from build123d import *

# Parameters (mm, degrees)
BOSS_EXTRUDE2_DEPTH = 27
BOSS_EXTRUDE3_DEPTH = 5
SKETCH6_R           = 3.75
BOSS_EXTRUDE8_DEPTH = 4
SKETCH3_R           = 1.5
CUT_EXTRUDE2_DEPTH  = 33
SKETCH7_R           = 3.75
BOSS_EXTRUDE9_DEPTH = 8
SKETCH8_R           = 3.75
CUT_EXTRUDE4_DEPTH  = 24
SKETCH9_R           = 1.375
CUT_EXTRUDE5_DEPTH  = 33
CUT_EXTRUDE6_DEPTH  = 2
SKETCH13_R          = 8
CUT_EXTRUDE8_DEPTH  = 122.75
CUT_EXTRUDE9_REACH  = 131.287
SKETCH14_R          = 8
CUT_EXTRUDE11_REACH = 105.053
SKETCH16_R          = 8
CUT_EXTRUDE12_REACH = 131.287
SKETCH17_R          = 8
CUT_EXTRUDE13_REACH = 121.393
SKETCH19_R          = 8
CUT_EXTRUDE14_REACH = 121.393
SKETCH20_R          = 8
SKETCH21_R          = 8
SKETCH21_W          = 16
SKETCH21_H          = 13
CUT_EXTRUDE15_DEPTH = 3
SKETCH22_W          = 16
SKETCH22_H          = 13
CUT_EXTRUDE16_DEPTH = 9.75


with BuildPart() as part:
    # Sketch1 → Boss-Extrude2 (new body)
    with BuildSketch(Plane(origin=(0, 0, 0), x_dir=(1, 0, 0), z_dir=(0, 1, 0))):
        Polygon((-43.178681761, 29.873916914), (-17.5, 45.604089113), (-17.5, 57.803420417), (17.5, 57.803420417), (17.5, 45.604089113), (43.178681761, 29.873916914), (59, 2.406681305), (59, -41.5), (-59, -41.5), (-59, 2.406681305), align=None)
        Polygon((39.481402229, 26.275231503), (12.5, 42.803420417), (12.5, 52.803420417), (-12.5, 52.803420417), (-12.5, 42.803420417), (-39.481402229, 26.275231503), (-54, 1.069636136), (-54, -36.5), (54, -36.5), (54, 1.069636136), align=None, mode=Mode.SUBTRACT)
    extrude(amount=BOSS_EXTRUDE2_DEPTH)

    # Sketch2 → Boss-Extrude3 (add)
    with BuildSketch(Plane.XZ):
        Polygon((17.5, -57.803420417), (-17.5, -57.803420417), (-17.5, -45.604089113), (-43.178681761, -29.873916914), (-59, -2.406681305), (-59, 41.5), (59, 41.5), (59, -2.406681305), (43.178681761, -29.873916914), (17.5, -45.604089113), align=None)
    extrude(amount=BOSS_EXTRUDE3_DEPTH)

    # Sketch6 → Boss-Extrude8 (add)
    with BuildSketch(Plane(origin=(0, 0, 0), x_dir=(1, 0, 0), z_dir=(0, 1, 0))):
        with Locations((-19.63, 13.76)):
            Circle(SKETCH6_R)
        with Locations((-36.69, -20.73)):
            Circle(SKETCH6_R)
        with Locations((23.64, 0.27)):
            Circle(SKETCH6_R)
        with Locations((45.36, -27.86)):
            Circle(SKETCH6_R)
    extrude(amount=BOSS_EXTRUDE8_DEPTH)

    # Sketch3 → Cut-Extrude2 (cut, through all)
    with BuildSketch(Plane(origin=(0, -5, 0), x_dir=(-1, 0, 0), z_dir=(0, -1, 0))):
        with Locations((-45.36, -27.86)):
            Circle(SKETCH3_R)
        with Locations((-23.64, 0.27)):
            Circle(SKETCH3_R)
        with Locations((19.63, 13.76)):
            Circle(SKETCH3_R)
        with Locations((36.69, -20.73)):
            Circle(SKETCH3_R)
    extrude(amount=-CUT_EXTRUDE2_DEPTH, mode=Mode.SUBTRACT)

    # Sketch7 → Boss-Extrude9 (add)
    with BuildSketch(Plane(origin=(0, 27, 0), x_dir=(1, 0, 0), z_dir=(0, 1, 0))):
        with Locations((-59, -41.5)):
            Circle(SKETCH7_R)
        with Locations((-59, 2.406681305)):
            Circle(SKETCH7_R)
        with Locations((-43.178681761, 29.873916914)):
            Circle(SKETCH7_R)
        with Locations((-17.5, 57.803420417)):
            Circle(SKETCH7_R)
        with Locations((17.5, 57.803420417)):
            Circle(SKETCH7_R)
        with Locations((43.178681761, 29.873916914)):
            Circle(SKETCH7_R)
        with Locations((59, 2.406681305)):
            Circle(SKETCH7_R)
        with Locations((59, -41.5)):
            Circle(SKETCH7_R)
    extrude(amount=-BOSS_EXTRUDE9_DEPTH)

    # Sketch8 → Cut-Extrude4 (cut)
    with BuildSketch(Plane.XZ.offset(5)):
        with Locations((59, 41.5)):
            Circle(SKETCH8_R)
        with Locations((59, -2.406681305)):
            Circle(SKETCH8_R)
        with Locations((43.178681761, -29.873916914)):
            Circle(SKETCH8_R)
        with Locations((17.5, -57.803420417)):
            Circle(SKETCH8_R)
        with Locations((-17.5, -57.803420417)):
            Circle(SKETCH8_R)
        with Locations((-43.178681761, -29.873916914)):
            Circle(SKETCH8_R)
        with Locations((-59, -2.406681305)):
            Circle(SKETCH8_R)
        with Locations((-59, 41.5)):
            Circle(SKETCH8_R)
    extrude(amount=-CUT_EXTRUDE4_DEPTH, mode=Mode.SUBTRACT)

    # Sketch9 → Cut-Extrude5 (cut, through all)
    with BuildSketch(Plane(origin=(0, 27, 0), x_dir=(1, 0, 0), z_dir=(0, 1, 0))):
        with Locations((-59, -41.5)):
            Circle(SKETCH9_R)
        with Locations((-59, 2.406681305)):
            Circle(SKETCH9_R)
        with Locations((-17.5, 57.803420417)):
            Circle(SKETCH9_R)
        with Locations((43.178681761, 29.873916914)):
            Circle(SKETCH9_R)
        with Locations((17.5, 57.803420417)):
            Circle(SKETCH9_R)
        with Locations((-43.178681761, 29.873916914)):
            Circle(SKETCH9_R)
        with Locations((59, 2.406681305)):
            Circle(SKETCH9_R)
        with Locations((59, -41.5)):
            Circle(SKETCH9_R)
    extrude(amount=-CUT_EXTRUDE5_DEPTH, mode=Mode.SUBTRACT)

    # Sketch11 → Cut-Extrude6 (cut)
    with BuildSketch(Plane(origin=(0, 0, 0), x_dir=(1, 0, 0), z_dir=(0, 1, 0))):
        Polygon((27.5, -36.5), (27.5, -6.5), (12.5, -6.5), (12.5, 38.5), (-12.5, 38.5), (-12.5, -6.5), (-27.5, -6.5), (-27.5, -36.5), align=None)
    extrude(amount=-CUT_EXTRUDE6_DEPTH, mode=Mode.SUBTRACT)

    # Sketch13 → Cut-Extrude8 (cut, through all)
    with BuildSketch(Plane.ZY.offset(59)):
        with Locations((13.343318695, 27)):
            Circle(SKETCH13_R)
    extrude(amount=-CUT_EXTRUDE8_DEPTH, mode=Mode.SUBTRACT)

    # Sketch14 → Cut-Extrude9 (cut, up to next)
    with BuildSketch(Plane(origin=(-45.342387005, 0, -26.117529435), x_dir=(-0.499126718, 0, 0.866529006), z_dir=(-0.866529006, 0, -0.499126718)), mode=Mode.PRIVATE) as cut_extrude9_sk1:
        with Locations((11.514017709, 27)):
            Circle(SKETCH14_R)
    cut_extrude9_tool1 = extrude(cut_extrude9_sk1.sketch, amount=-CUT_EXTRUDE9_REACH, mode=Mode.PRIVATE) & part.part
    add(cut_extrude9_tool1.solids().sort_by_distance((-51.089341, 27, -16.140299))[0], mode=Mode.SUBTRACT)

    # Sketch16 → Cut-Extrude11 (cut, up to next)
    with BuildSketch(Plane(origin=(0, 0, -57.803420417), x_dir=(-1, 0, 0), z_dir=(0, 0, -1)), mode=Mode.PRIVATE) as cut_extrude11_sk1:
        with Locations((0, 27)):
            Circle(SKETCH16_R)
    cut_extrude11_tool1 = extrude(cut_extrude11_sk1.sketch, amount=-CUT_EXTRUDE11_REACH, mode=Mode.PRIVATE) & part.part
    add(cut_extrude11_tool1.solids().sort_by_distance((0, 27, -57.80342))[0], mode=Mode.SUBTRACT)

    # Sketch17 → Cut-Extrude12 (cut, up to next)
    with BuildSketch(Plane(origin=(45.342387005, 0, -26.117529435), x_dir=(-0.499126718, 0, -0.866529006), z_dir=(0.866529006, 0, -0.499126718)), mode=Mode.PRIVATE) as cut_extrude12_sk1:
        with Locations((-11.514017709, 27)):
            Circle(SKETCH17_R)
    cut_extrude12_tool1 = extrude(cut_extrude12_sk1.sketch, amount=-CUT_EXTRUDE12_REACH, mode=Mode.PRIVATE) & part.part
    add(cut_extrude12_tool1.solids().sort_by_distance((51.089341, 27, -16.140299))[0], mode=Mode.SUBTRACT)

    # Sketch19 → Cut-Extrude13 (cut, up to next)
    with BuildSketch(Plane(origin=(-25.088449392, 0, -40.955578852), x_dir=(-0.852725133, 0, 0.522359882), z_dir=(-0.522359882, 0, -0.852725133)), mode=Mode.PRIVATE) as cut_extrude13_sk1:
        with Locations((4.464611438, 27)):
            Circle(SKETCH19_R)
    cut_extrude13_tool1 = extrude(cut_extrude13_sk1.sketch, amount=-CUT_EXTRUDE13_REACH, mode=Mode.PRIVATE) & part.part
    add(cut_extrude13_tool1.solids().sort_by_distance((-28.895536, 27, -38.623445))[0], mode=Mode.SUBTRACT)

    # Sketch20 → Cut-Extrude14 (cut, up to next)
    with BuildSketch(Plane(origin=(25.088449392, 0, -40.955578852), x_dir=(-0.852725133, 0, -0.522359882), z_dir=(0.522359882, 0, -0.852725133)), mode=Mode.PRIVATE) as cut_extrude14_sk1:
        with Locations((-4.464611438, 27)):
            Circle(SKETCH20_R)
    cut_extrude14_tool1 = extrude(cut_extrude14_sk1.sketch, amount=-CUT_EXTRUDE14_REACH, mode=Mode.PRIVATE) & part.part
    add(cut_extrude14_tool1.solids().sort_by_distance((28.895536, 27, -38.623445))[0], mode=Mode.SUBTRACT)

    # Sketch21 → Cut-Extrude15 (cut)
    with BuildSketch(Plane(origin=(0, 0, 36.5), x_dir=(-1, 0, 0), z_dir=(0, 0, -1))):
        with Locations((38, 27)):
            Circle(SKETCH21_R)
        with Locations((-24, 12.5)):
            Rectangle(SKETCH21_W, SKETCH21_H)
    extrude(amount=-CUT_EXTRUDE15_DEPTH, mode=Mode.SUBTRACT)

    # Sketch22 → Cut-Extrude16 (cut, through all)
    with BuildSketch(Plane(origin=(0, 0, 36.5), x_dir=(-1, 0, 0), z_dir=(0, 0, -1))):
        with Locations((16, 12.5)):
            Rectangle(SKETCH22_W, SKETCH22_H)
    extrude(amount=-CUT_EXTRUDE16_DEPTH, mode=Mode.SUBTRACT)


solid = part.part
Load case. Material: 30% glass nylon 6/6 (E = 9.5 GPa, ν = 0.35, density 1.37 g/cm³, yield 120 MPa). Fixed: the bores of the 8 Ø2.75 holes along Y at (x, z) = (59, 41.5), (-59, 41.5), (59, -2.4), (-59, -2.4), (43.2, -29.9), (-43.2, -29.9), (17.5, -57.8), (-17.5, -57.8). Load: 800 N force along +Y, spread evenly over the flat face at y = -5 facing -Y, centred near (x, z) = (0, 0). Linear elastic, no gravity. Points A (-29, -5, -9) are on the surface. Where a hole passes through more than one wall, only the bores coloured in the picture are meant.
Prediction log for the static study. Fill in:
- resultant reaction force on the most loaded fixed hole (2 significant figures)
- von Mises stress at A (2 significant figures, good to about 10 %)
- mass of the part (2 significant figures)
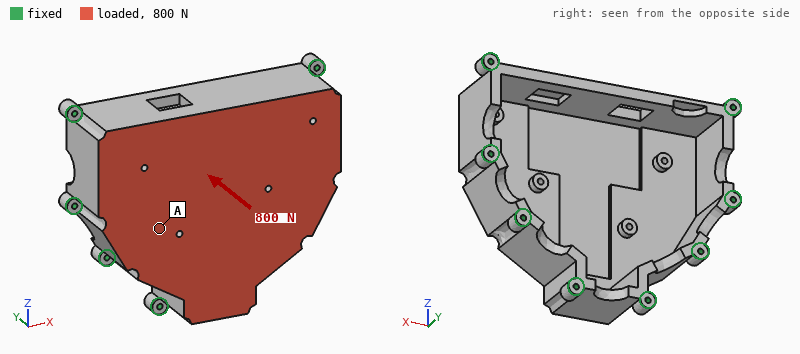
210 N
2.8 MPa
120 g
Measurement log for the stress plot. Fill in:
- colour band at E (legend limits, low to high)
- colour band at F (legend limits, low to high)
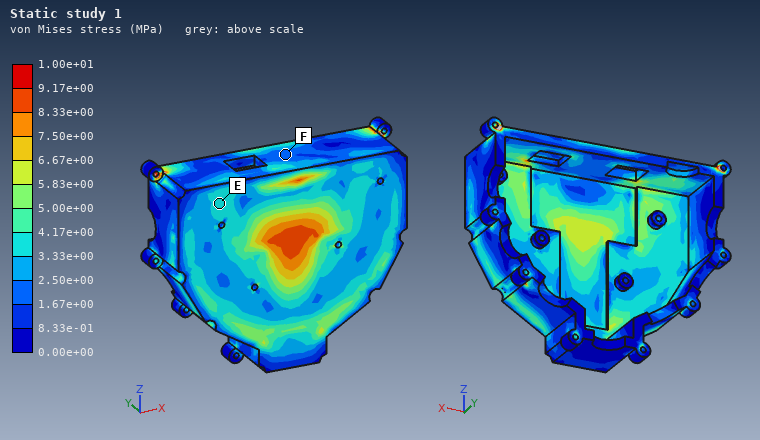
3.33e+00 to 4.17e+00 MPa
1.67e+00 to 2.50e+00 MPa
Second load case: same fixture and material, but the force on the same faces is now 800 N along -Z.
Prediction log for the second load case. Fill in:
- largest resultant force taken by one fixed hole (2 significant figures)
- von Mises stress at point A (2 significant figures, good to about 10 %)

170 N
0.86 MPa
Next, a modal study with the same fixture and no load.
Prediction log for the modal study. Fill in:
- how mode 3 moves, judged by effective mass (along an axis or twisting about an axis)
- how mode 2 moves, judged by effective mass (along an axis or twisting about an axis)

along X
along Y
